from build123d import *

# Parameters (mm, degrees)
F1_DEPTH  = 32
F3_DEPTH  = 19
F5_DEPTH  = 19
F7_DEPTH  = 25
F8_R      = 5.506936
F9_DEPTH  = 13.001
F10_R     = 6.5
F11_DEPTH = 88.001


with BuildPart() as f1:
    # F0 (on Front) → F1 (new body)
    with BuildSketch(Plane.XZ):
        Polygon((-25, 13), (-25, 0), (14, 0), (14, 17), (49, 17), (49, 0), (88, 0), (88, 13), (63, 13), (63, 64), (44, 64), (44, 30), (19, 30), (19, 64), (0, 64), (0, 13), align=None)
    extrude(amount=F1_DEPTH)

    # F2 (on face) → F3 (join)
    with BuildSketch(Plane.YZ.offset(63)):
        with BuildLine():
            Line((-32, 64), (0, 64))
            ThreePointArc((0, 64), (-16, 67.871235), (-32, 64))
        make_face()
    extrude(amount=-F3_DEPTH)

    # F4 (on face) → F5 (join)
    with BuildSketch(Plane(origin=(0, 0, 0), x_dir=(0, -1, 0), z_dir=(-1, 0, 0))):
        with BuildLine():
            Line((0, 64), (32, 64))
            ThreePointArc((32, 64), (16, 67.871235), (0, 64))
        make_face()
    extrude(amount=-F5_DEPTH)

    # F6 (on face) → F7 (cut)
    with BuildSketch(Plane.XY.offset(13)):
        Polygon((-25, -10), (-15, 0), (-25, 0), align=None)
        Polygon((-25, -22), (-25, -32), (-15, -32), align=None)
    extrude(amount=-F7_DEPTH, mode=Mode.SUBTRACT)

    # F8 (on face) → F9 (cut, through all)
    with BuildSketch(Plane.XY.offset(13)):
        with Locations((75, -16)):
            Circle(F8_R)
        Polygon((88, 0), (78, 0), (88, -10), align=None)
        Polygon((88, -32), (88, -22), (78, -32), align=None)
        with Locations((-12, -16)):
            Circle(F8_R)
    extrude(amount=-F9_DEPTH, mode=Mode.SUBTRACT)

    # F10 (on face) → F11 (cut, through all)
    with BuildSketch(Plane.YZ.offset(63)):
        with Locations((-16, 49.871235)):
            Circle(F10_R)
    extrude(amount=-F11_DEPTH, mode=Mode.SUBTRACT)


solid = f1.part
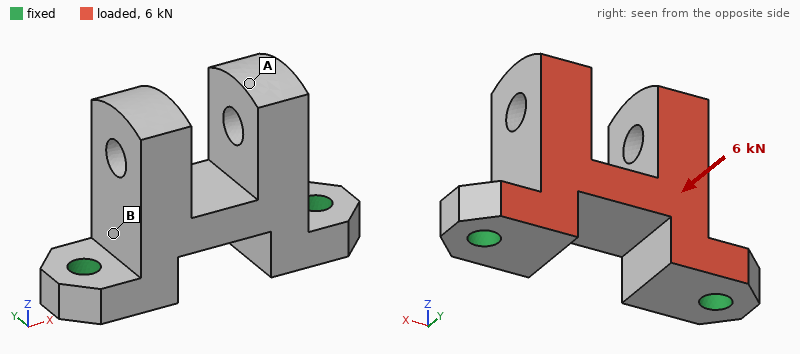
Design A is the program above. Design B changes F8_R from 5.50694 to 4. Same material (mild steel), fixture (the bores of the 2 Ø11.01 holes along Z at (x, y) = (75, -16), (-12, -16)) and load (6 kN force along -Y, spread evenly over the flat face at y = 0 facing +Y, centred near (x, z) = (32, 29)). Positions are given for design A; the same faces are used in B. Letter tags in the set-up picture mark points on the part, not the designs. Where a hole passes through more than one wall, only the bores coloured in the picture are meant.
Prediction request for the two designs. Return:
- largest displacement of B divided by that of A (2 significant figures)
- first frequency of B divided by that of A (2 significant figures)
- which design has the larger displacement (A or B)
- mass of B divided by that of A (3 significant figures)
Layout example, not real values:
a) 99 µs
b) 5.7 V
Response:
a) 1.2
b) 0.90
c) B
d) 1.01
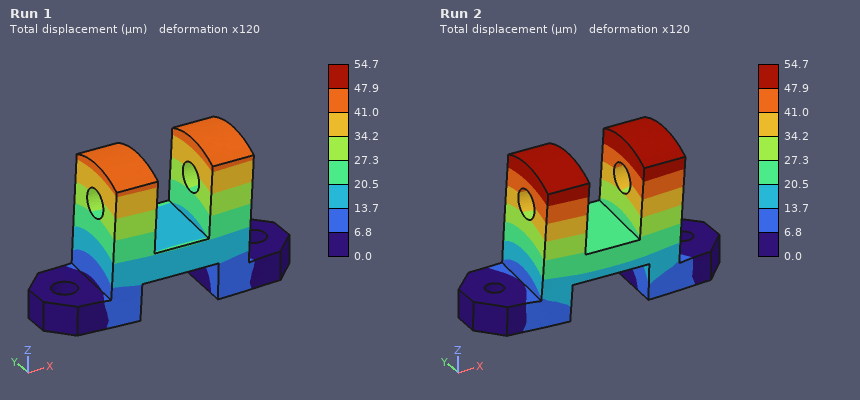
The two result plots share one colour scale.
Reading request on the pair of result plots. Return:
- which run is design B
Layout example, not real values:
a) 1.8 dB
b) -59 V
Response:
a) Run 2
